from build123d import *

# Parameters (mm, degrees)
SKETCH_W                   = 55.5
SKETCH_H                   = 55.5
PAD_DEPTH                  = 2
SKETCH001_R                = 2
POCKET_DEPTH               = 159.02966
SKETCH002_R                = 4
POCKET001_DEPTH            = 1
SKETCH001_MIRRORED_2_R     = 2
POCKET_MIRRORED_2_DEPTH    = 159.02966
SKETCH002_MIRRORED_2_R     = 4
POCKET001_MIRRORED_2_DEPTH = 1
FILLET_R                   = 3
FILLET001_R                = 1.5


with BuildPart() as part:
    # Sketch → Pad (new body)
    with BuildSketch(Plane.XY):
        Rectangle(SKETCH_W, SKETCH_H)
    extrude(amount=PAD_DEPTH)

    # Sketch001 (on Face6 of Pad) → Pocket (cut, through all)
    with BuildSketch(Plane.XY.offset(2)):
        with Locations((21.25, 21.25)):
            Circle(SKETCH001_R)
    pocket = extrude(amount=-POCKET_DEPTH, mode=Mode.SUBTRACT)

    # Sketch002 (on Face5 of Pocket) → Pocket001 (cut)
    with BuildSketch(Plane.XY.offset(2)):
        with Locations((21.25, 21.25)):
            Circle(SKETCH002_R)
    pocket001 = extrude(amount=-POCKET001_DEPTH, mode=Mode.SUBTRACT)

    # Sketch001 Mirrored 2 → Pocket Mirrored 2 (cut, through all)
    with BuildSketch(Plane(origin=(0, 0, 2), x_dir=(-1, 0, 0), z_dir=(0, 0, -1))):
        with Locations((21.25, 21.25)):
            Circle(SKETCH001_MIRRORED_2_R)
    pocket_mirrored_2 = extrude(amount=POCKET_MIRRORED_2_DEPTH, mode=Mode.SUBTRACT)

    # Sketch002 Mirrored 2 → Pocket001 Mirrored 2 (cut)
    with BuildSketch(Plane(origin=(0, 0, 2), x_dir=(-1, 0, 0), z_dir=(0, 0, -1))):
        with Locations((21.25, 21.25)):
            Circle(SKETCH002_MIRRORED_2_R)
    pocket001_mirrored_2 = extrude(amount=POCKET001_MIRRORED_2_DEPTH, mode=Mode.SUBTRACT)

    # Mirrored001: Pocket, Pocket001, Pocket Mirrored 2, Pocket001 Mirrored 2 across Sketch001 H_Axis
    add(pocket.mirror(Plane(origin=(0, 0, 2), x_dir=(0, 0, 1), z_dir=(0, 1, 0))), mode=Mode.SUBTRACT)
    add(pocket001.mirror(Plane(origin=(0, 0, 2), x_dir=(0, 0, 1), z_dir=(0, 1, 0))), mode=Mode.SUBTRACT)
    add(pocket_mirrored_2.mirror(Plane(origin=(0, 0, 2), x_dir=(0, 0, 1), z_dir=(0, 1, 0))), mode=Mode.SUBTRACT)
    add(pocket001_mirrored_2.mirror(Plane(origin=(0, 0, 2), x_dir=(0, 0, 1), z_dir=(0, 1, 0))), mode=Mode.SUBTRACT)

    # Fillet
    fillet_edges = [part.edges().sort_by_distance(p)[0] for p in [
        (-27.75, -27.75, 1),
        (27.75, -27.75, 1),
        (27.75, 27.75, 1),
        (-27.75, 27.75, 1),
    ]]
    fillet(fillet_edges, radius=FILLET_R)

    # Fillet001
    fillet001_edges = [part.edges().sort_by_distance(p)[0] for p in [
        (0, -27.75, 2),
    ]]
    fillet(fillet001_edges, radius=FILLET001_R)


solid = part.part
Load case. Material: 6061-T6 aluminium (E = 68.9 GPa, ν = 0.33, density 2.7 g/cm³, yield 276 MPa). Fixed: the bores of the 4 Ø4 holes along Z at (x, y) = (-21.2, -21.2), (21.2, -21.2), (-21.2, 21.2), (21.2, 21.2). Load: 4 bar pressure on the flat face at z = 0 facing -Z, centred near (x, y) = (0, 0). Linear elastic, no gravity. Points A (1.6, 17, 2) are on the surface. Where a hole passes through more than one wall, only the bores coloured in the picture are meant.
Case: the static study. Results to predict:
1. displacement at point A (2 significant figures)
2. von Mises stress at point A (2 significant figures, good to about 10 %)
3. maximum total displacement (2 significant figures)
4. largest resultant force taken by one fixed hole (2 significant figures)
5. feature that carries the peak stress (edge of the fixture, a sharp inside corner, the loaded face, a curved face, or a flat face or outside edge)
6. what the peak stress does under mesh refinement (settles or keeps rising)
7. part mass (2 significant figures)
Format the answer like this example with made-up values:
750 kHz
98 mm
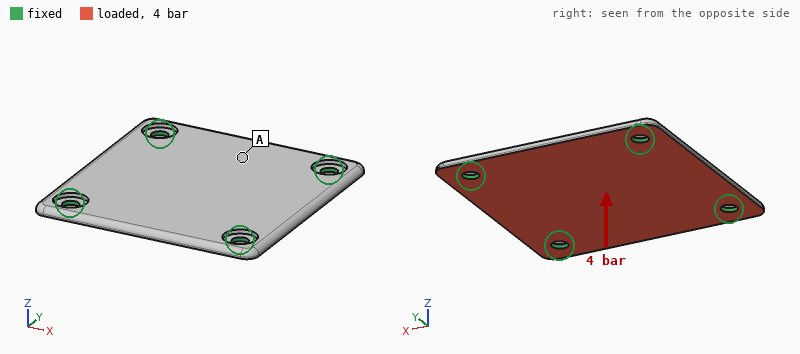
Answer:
0.15 mm
67 MPa
0.22 mm
590 N
edge of the fixture
keeps rising
16 g
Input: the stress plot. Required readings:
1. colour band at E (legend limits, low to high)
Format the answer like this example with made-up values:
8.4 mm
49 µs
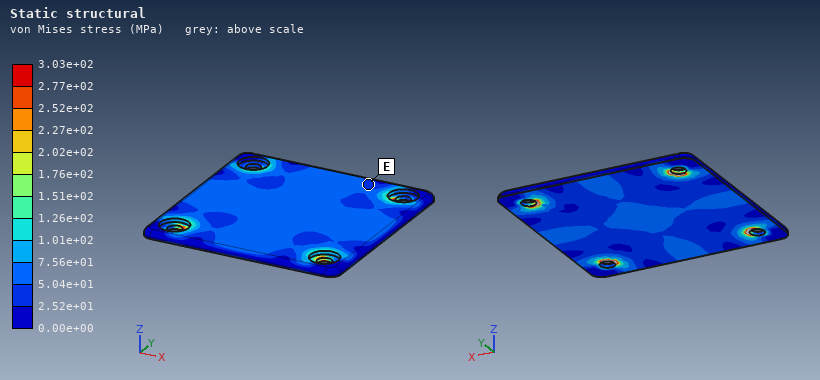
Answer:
2.52e+01 to 5.04e+01 MPa
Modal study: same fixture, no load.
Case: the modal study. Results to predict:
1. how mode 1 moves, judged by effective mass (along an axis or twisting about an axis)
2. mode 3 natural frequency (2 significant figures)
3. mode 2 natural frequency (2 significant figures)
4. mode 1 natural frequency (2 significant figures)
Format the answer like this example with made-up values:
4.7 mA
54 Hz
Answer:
along Z
5600 Hz
5600 Hz
3600 Hz
